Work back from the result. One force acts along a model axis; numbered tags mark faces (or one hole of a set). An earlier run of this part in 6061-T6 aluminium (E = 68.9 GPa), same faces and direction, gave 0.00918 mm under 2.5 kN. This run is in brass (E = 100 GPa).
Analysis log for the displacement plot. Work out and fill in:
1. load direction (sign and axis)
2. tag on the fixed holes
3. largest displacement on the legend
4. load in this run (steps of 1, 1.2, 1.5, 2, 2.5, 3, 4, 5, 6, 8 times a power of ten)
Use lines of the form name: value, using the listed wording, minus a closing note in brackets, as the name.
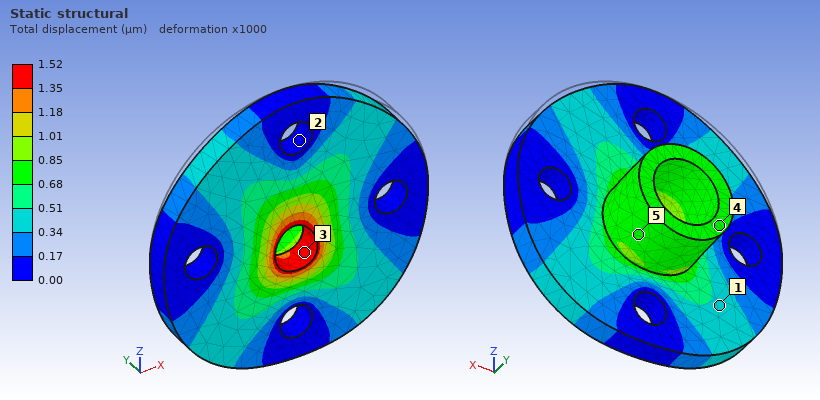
load direction: -Z
tag on the fixed holes: 2
largest displacement on the legend: 1.52 µm
load in this run: 600 N
